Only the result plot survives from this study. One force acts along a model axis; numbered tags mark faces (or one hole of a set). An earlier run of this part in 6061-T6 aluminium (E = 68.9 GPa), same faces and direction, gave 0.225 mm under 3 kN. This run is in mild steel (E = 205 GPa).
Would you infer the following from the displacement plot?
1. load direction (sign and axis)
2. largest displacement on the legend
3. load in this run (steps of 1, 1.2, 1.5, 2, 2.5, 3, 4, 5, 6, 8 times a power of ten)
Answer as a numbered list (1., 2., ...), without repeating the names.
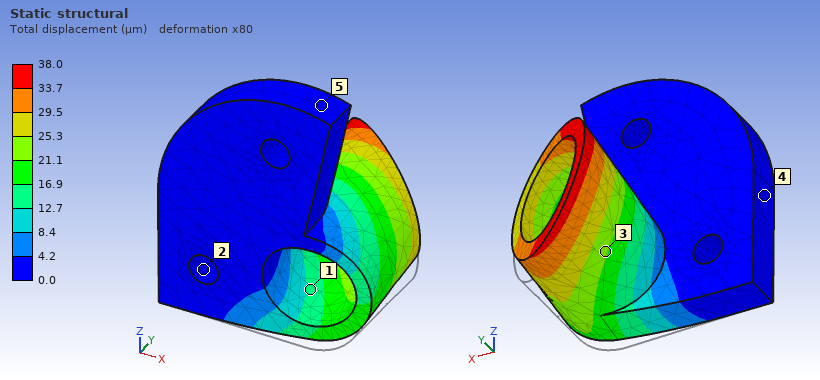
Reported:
1. +Z
2. 38.0 µm
3. 1.5 kN
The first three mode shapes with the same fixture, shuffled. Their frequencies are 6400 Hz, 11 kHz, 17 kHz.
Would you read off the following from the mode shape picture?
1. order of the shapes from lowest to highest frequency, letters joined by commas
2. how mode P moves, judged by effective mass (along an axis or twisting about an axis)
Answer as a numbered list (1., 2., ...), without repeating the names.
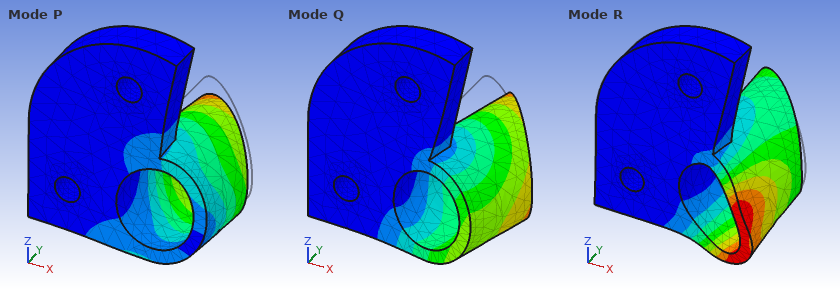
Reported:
1. Q, P, R
2. along Z
